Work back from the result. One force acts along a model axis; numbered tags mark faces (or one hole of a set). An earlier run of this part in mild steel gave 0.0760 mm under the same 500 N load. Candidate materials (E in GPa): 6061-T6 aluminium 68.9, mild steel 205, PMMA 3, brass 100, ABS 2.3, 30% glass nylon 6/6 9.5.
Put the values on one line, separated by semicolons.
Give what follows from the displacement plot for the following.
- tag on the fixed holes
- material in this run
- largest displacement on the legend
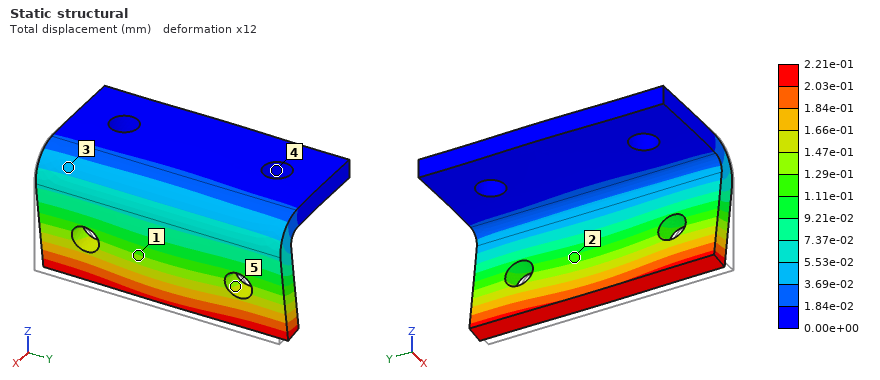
4; 6061-T6 aluminium; 2.21e-01 mm
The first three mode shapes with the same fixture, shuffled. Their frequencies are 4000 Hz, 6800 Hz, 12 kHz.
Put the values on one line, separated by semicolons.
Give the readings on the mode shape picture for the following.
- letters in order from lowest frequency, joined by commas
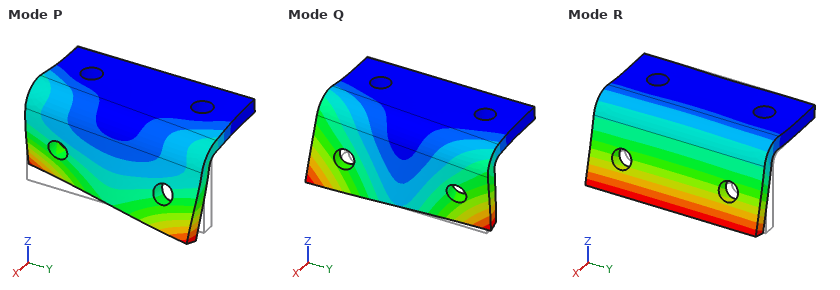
R, Q, P
